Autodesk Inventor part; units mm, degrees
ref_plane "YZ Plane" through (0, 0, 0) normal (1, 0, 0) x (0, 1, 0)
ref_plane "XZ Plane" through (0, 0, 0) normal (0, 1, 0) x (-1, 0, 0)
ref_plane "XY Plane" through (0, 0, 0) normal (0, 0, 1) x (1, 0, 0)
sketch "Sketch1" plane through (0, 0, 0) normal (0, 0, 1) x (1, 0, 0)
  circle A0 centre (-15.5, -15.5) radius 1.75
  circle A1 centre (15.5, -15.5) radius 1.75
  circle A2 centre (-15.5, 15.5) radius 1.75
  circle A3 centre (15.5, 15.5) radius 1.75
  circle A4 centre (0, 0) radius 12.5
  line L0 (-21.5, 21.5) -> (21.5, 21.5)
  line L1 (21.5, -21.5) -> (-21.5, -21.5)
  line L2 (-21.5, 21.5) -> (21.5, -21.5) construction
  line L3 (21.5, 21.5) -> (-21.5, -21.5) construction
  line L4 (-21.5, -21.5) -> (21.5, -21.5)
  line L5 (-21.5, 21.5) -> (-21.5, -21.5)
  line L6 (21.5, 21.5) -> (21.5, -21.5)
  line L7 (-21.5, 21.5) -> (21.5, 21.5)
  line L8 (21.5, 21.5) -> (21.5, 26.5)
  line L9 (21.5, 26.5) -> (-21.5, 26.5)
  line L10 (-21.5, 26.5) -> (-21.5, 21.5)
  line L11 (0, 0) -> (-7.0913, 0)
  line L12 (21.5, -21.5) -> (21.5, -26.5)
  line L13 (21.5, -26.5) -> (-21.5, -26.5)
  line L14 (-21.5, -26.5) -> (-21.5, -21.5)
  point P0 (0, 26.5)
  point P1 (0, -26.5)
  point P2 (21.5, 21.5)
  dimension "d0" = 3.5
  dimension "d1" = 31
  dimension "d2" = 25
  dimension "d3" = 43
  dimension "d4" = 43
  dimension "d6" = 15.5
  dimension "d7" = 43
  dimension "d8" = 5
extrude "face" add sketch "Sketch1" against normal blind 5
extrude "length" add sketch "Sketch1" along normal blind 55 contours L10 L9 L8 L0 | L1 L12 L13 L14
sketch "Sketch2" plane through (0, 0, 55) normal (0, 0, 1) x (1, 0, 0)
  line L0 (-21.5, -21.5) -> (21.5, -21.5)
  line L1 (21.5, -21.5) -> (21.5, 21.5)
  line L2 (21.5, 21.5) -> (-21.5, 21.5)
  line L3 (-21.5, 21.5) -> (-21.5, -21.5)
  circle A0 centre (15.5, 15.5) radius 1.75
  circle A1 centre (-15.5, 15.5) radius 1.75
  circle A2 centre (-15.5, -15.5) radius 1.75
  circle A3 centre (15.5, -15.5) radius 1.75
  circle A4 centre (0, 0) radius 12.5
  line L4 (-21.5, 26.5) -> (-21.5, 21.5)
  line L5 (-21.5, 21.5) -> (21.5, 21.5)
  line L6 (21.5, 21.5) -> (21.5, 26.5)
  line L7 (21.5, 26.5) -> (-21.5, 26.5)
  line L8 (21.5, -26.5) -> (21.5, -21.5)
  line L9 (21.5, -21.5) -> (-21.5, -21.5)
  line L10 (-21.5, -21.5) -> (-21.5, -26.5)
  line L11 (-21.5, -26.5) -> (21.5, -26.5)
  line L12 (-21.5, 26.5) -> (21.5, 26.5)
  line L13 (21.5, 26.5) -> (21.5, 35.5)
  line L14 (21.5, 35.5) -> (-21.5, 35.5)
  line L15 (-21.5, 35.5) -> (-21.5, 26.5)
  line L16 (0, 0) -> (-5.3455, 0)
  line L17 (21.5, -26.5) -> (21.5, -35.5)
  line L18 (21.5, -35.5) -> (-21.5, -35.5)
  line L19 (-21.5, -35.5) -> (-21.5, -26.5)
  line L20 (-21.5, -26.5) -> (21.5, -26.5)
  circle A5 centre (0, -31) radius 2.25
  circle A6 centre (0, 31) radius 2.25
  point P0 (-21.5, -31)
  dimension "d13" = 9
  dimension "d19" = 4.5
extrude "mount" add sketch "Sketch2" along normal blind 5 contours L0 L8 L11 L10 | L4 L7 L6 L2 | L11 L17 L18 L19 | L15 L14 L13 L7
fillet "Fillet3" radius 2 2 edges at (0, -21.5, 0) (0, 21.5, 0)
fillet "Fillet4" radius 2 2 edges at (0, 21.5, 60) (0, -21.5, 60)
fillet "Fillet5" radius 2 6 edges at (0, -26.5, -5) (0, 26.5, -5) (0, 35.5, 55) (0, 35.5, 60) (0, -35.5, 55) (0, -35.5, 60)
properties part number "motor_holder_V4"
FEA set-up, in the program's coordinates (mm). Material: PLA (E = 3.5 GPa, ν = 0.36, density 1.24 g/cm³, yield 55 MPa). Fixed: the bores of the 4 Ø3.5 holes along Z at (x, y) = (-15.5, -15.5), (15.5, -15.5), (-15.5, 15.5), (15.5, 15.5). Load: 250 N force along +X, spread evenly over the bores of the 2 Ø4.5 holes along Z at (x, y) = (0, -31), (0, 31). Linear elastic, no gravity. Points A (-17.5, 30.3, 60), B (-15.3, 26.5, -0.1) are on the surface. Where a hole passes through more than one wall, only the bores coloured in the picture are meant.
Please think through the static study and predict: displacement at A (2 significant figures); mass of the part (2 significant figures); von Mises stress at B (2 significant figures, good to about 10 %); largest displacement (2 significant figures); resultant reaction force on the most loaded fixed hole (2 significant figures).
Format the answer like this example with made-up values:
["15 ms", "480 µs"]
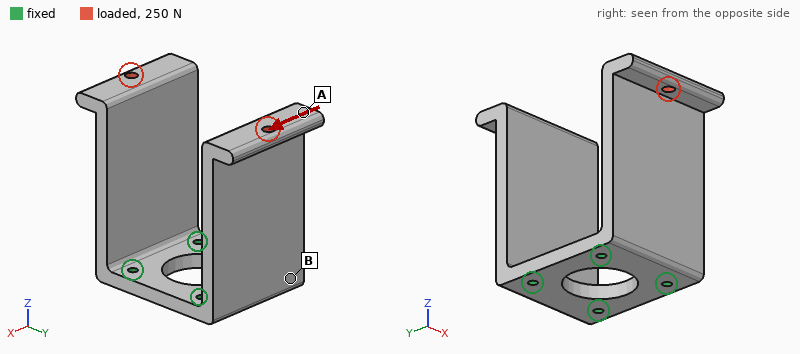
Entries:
["0.47 mm", "47 g", "3.7 MPa", "0.54 mm", "240 N"]
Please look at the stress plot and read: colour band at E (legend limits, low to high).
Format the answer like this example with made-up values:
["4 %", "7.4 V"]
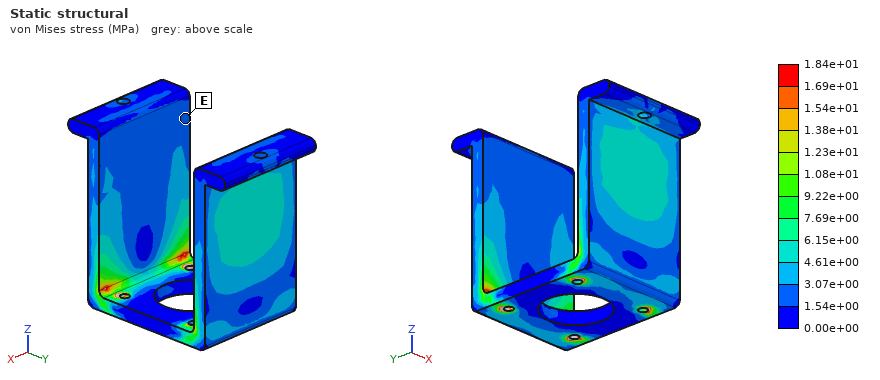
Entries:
["1.54e+00 to 3.07e+00 MPa"]
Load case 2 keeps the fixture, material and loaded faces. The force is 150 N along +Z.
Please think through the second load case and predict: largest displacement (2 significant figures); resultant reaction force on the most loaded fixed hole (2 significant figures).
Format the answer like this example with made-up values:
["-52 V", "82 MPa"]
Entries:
["0.96 mm", "38 N"]
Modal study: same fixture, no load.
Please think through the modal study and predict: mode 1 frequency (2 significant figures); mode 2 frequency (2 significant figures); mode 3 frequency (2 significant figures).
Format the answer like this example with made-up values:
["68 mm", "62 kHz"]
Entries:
["240 Hz", "240 Hz", "890 Hz"]
